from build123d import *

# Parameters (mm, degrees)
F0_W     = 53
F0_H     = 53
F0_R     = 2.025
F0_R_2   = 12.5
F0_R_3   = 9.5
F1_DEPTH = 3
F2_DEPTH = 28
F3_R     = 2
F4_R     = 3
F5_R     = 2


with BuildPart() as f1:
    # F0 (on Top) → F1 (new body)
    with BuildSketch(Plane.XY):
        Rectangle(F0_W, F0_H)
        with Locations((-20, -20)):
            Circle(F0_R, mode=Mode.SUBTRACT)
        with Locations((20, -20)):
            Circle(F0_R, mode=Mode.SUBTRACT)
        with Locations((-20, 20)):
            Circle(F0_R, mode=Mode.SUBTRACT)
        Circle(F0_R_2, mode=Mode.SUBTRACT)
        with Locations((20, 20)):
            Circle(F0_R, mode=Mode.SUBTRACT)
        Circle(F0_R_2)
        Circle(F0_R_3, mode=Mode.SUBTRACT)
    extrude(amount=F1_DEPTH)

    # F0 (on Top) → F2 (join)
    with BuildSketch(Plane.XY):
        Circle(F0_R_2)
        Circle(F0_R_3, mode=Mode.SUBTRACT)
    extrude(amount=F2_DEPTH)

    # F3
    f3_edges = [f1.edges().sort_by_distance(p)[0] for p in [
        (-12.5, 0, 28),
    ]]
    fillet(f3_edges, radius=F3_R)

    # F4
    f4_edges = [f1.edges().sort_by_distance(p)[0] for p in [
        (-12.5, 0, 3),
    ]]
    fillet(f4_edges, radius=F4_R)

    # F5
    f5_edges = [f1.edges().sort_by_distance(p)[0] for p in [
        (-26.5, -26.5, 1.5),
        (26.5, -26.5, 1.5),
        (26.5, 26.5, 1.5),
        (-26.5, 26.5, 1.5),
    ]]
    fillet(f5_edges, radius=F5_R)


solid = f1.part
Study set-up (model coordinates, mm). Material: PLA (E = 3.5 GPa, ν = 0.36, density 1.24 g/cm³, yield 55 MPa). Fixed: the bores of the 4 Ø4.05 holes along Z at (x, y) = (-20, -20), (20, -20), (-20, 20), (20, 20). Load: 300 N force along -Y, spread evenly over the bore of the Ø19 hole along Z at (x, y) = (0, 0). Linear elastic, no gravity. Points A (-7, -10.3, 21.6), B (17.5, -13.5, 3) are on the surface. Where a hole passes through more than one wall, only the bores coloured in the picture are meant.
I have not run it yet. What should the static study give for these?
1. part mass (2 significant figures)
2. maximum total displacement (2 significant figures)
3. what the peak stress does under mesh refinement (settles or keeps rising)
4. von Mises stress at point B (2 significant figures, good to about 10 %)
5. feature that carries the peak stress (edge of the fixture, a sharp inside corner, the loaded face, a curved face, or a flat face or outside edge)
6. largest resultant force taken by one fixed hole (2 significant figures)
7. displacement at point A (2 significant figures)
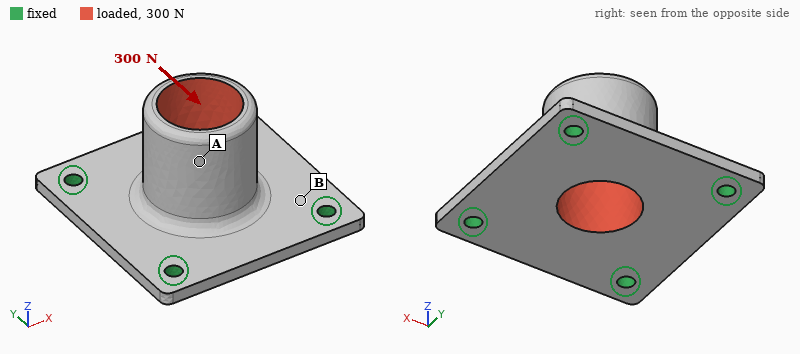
16 g
0.29 mm
keeps rising
5.3 MPa
edge of the fixture
100 N
0.23 mm
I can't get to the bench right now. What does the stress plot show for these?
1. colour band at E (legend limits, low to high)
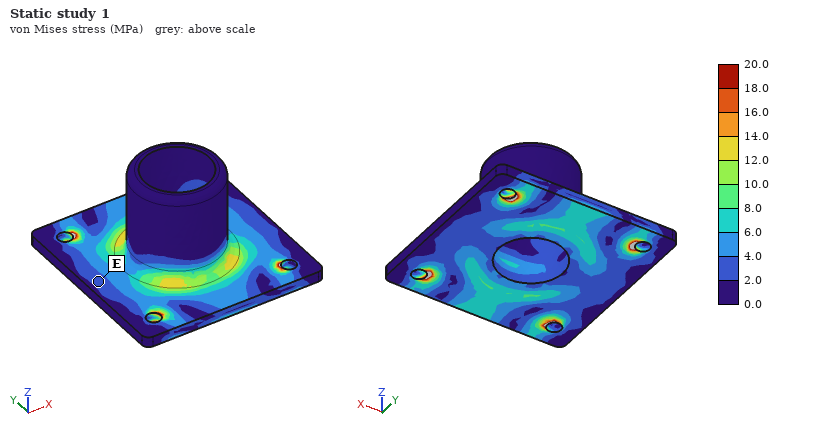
2.0 to 4.0 MPa
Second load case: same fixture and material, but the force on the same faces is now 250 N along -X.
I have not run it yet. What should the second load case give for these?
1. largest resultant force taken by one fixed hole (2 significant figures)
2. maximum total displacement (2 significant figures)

84 N
0.24 mm
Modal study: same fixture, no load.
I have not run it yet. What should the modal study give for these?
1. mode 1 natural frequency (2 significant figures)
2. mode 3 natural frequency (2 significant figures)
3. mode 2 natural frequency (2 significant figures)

2000 Hz
2000 Hz
2000 Hz
